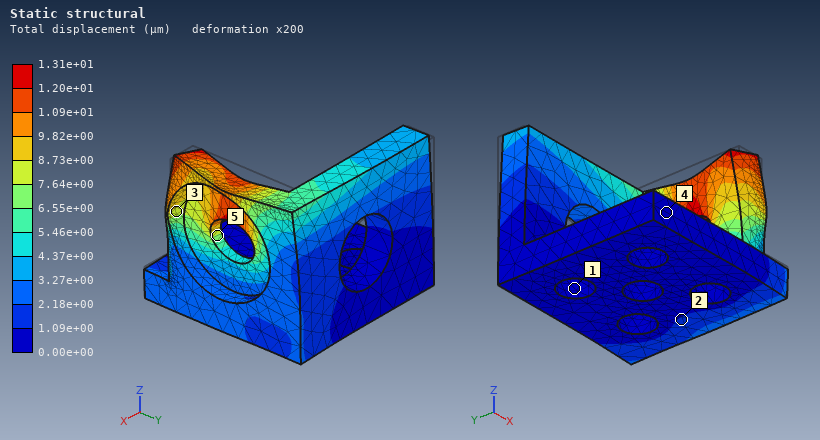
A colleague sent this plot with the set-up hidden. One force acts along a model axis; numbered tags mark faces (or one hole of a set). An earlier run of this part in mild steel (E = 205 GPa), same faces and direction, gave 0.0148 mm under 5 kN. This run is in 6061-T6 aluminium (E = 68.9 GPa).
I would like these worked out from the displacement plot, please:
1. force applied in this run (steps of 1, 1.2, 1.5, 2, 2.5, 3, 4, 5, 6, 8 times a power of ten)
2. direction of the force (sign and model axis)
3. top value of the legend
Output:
1.5 kN
-Z
1.31e+01 µm
